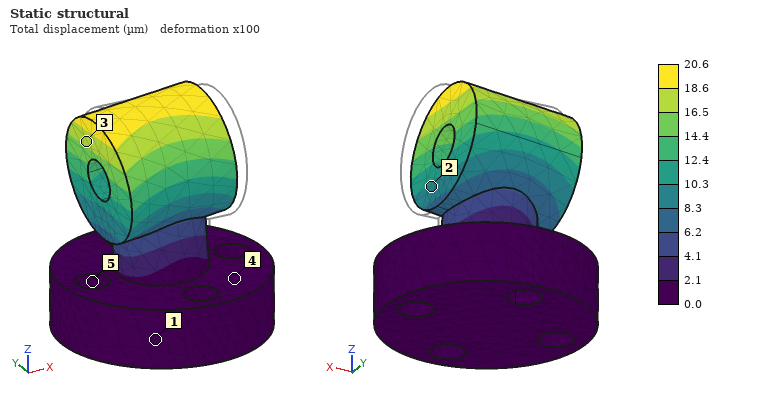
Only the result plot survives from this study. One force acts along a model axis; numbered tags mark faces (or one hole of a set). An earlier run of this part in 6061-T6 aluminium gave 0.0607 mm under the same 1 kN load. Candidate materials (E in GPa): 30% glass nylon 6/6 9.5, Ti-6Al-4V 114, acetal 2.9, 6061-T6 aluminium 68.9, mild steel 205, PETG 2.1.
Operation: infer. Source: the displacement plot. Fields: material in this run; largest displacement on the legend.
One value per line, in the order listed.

mild steel
20.6 µm
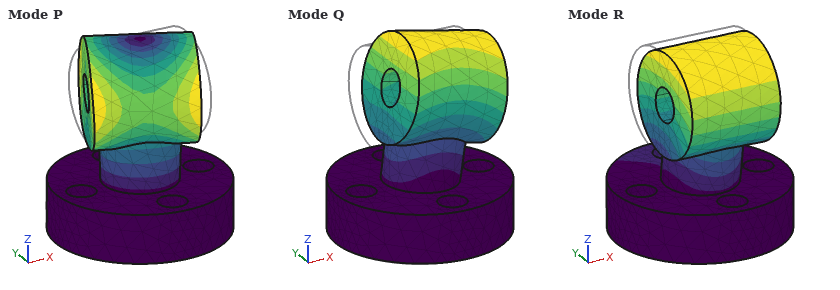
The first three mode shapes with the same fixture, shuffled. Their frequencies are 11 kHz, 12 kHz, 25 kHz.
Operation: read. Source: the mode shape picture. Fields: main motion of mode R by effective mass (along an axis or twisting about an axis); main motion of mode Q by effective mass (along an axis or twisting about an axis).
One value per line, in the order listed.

along Y
along X
